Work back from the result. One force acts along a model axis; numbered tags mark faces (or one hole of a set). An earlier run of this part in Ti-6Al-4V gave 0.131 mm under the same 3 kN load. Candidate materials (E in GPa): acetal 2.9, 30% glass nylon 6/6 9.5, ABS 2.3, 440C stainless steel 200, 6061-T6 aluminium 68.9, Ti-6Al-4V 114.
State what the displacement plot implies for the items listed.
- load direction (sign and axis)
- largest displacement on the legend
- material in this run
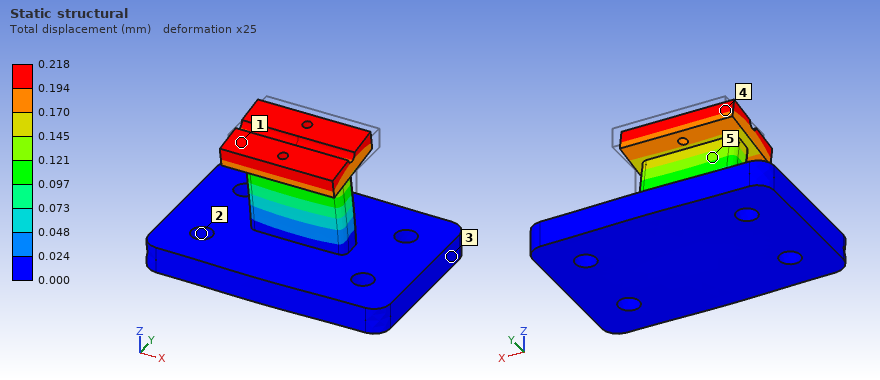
-Y
0.218 mm
6061-T6 aluminium
